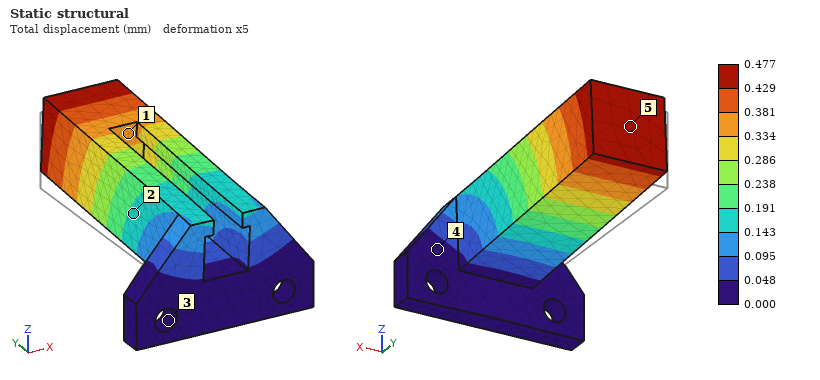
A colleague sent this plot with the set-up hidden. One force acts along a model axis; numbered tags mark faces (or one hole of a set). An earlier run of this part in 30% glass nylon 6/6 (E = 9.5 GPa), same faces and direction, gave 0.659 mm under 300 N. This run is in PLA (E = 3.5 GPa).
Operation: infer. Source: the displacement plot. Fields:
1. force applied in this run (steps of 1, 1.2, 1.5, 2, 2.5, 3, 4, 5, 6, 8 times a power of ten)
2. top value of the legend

80 N
0.477 mm
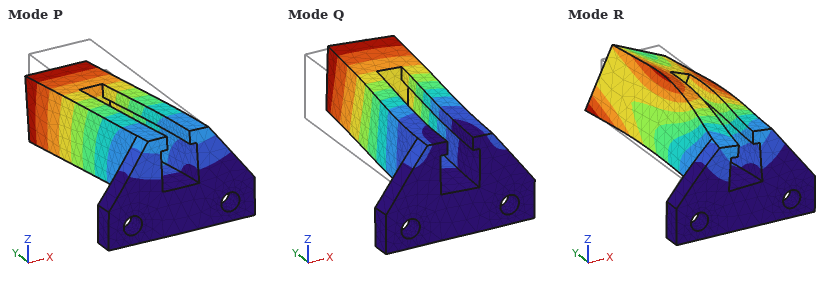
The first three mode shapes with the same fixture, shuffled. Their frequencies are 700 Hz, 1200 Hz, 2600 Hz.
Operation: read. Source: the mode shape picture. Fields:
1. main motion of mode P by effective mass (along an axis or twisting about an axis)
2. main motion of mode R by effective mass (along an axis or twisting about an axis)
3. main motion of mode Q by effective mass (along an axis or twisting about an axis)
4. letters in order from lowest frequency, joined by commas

along Z
twisting about Y
along X
P, Q, R
